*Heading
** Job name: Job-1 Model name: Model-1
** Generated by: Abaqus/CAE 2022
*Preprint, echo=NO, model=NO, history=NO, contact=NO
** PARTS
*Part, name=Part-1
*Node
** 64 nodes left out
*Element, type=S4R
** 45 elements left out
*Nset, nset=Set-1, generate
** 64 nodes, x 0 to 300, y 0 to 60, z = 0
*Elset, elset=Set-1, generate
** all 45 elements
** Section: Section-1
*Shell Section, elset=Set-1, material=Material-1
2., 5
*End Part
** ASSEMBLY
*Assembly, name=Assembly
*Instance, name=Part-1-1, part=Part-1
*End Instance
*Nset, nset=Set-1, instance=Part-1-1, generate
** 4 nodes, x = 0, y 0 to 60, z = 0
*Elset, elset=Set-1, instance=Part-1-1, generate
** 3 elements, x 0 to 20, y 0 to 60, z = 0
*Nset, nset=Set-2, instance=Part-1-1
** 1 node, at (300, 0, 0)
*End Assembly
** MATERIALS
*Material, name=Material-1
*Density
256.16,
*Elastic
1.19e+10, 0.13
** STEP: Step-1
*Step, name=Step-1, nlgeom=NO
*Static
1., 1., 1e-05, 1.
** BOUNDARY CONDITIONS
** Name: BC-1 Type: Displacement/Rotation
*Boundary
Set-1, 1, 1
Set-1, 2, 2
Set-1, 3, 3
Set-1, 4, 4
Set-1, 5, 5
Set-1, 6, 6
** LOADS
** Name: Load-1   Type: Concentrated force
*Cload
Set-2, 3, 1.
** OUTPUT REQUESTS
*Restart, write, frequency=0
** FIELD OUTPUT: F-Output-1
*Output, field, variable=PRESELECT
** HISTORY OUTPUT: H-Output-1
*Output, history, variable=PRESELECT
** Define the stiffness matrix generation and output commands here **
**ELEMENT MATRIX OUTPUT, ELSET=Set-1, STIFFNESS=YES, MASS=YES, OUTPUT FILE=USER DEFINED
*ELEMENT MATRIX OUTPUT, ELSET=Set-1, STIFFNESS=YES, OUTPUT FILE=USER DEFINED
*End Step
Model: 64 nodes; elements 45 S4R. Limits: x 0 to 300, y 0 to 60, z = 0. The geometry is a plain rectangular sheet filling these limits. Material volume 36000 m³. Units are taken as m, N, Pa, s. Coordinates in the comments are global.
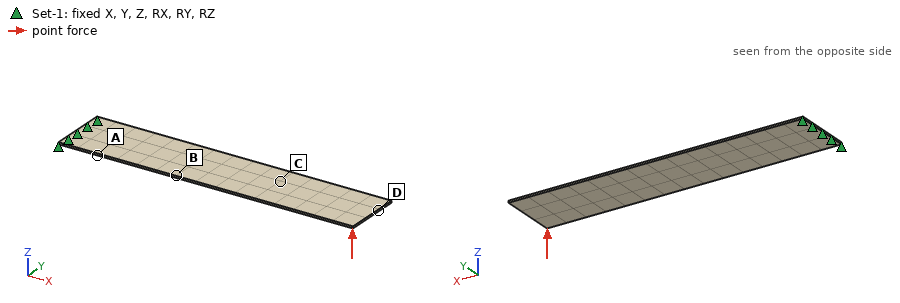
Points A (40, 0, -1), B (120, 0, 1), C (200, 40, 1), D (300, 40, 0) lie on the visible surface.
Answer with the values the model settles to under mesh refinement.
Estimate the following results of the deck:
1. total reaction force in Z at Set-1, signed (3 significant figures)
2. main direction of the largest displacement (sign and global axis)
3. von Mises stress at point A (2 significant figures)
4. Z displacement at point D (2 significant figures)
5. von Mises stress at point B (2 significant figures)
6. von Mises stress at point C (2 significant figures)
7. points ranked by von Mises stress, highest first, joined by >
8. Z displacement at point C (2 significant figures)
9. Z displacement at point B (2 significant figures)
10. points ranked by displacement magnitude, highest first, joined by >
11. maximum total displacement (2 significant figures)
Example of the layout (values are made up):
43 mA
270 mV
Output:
-1.00 N
+Z
6.6 Pa
1.9e-05 m
4.5 Pa
2.6 Pa
A > B > C > D
9.7e-06 m
4.0e-06 m
D > C > B > A
1.9e-05 m
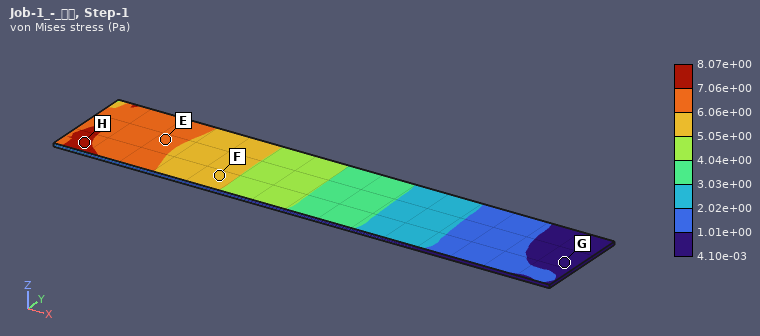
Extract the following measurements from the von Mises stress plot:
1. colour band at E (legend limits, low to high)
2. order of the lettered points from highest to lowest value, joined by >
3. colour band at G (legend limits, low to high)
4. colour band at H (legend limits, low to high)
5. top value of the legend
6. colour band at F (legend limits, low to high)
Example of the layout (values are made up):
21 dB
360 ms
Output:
6.06e+00 to 7.06e+00 Pa
H > E > F > G
4.10e-03 to 1.01e+00 Pa
7.06e+00 to 8.07e+00 Pa
8.07e+00 Pa
5.05e+00 to 6.06e+00 Pa
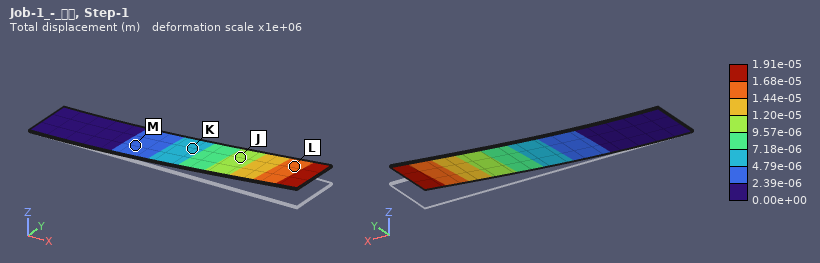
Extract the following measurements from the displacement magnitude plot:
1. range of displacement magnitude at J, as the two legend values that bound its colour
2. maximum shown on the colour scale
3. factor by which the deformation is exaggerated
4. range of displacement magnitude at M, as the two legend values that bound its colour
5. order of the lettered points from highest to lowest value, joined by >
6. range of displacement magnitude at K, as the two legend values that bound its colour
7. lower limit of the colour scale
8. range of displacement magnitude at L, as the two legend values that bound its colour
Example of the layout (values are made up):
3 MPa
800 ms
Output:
9.57e-06 to 1.20e-05 m
1.91e-05 m
1e+06
2.39e-06 to 4.79e-06 m
L > J > K > M
4.79e-06 to 7.18e-06 m
0.00e+00 m
1.44e-05 to 1.68e-05 m
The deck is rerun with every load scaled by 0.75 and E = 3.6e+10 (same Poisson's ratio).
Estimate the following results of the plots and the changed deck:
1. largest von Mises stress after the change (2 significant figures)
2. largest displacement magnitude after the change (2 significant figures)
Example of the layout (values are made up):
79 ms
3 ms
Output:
6.1 Pa
4.7e-06 m
